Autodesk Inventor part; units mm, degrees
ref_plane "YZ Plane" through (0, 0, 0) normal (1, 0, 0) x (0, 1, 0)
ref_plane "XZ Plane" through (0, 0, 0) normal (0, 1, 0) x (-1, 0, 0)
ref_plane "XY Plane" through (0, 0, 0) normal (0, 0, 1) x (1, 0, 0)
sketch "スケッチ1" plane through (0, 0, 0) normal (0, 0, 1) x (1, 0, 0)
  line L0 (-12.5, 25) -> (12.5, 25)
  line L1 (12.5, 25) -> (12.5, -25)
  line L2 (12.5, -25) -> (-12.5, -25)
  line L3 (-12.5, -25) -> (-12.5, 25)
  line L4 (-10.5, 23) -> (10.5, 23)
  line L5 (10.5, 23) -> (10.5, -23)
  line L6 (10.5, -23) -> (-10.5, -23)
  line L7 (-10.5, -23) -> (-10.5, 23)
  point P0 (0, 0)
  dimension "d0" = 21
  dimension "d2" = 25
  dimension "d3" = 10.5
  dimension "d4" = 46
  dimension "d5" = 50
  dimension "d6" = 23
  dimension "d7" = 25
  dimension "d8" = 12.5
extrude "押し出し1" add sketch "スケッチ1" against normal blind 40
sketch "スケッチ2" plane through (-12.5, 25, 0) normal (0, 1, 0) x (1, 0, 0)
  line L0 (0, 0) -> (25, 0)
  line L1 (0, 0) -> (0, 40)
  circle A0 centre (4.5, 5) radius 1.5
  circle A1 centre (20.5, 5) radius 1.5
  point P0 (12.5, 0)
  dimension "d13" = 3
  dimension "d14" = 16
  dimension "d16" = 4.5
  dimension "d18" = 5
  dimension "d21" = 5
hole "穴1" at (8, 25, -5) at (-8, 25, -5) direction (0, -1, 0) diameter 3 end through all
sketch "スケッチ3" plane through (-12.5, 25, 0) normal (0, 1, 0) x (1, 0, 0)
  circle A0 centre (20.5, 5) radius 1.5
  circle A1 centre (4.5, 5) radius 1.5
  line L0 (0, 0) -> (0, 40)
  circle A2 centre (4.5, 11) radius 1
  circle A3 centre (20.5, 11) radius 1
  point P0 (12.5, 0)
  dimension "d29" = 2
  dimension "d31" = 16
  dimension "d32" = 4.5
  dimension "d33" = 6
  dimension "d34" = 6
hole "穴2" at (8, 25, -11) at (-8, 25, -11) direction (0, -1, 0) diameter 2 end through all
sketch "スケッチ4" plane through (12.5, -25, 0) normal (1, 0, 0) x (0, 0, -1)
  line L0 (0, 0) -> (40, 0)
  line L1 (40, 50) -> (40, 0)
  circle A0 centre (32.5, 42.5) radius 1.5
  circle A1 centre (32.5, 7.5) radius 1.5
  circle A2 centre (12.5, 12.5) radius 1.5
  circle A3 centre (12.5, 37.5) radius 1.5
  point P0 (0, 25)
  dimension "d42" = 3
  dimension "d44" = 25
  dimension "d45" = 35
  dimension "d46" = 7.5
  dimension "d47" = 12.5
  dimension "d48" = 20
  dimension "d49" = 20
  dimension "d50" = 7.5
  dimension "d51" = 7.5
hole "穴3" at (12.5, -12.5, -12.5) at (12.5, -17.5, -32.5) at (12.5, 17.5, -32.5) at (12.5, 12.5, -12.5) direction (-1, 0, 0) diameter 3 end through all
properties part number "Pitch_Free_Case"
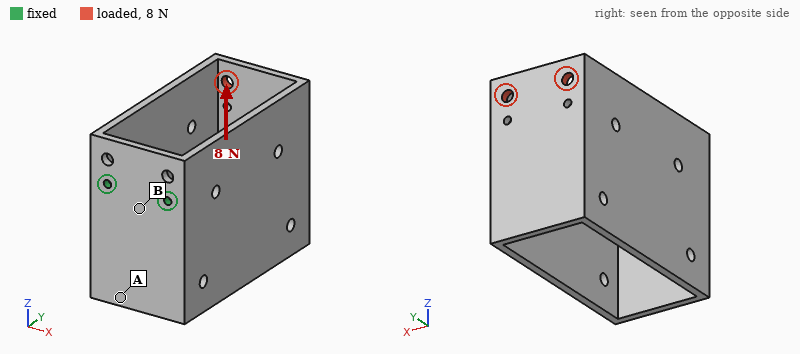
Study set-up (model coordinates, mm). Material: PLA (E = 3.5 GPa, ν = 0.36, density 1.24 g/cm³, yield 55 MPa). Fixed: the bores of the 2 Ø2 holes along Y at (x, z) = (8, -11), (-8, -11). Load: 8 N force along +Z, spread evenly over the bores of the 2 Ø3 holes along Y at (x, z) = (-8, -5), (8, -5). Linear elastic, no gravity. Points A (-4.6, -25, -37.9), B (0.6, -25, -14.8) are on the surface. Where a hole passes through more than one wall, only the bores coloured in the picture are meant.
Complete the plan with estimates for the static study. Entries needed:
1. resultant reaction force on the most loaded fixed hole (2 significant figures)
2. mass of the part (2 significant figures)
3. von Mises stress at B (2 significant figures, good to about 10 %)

4.0 N
14 g
2.6 MPa
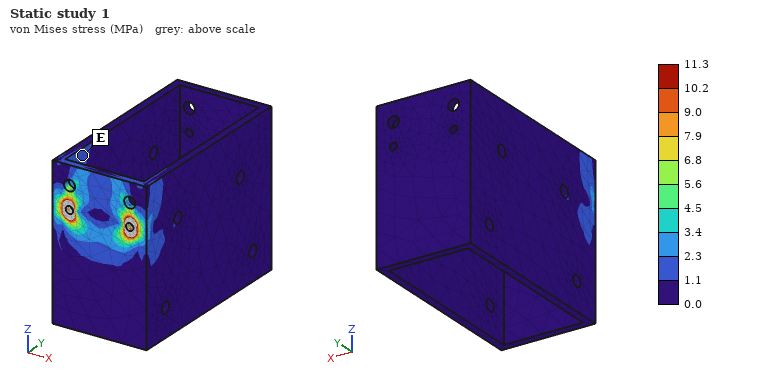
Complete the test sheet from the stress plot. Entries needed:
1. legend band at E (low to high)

1.1 to 2.3 MPa
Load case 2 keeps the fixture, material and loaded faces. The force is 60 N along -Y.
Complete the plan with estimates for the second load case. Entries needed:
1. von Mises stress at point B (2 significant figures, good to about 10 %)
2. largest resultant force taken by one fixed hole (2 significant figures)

2.3 MPa
30 N
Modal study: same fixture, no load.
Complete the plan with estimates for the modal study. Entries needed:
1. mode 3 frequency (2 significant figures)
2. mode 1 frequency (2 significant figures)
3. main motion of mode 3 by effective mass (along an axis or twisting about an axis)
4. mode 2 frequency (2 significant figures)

600 Hz
230 Hz
twisting about Y
230 Hz
